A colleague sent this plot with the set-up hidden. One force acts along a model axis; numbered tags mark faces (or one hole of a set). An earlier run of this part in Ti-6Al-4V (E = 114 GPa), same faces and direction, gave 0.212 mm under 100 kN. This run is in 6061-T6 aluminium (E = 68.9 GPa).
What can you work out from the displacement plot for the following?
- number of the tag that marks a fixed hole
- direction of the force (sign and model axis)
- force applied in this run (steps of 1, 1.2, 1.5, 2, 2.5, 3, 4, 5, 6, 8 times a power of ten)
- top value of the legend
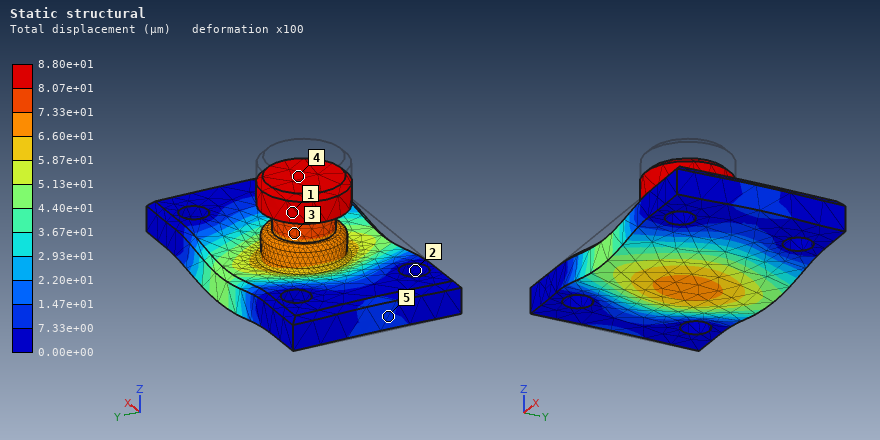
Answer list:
2
-Z
25 kN
8.80e+01 µm
